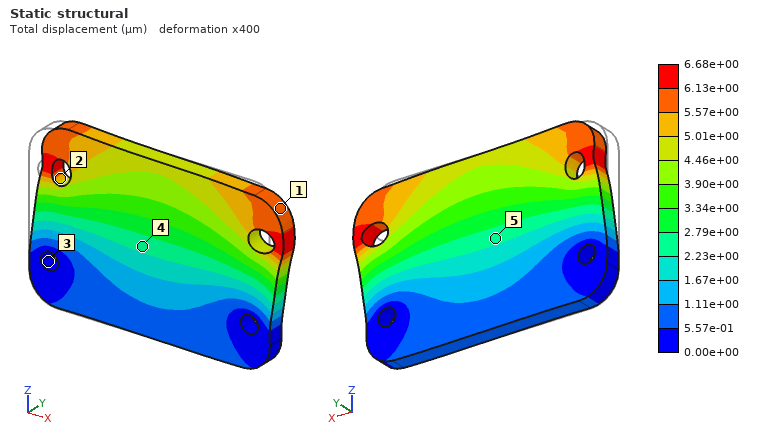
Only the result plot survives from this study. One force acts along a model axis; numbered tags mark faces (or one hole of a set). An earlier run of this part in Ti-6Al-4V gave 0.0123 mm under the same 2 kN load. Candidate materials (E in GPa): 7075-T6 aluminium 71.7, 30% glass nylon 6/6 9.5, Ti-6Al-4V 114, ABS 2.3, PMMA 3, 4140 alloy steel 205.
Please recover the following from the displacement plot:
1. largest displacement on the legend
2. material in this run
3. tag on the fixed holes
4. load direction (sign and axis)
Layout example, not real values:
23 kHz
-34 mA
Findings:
6.68e+00 µm
4140 alloy steel
3
+X
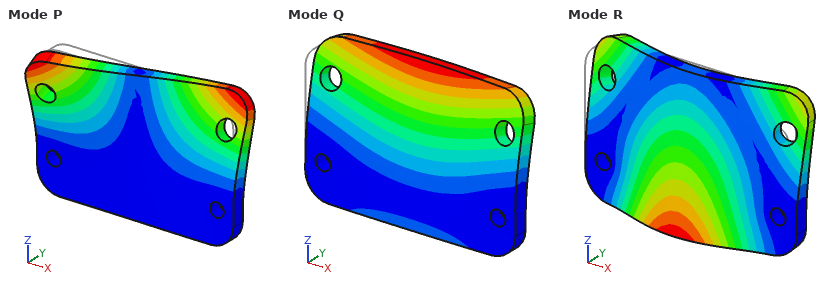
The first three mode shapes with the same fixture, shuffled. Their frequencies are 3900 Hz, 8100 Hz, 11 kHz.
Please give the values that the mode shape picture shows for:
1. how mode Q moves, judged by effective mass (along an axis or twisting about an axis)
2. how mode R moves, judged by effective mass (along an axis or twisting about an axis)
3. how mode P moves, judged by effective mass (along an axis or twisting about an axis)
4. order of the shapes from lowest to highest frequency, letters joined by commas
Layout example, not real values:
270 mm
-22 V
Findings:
along Y
along Y
twisting about Z
Q, P, R
